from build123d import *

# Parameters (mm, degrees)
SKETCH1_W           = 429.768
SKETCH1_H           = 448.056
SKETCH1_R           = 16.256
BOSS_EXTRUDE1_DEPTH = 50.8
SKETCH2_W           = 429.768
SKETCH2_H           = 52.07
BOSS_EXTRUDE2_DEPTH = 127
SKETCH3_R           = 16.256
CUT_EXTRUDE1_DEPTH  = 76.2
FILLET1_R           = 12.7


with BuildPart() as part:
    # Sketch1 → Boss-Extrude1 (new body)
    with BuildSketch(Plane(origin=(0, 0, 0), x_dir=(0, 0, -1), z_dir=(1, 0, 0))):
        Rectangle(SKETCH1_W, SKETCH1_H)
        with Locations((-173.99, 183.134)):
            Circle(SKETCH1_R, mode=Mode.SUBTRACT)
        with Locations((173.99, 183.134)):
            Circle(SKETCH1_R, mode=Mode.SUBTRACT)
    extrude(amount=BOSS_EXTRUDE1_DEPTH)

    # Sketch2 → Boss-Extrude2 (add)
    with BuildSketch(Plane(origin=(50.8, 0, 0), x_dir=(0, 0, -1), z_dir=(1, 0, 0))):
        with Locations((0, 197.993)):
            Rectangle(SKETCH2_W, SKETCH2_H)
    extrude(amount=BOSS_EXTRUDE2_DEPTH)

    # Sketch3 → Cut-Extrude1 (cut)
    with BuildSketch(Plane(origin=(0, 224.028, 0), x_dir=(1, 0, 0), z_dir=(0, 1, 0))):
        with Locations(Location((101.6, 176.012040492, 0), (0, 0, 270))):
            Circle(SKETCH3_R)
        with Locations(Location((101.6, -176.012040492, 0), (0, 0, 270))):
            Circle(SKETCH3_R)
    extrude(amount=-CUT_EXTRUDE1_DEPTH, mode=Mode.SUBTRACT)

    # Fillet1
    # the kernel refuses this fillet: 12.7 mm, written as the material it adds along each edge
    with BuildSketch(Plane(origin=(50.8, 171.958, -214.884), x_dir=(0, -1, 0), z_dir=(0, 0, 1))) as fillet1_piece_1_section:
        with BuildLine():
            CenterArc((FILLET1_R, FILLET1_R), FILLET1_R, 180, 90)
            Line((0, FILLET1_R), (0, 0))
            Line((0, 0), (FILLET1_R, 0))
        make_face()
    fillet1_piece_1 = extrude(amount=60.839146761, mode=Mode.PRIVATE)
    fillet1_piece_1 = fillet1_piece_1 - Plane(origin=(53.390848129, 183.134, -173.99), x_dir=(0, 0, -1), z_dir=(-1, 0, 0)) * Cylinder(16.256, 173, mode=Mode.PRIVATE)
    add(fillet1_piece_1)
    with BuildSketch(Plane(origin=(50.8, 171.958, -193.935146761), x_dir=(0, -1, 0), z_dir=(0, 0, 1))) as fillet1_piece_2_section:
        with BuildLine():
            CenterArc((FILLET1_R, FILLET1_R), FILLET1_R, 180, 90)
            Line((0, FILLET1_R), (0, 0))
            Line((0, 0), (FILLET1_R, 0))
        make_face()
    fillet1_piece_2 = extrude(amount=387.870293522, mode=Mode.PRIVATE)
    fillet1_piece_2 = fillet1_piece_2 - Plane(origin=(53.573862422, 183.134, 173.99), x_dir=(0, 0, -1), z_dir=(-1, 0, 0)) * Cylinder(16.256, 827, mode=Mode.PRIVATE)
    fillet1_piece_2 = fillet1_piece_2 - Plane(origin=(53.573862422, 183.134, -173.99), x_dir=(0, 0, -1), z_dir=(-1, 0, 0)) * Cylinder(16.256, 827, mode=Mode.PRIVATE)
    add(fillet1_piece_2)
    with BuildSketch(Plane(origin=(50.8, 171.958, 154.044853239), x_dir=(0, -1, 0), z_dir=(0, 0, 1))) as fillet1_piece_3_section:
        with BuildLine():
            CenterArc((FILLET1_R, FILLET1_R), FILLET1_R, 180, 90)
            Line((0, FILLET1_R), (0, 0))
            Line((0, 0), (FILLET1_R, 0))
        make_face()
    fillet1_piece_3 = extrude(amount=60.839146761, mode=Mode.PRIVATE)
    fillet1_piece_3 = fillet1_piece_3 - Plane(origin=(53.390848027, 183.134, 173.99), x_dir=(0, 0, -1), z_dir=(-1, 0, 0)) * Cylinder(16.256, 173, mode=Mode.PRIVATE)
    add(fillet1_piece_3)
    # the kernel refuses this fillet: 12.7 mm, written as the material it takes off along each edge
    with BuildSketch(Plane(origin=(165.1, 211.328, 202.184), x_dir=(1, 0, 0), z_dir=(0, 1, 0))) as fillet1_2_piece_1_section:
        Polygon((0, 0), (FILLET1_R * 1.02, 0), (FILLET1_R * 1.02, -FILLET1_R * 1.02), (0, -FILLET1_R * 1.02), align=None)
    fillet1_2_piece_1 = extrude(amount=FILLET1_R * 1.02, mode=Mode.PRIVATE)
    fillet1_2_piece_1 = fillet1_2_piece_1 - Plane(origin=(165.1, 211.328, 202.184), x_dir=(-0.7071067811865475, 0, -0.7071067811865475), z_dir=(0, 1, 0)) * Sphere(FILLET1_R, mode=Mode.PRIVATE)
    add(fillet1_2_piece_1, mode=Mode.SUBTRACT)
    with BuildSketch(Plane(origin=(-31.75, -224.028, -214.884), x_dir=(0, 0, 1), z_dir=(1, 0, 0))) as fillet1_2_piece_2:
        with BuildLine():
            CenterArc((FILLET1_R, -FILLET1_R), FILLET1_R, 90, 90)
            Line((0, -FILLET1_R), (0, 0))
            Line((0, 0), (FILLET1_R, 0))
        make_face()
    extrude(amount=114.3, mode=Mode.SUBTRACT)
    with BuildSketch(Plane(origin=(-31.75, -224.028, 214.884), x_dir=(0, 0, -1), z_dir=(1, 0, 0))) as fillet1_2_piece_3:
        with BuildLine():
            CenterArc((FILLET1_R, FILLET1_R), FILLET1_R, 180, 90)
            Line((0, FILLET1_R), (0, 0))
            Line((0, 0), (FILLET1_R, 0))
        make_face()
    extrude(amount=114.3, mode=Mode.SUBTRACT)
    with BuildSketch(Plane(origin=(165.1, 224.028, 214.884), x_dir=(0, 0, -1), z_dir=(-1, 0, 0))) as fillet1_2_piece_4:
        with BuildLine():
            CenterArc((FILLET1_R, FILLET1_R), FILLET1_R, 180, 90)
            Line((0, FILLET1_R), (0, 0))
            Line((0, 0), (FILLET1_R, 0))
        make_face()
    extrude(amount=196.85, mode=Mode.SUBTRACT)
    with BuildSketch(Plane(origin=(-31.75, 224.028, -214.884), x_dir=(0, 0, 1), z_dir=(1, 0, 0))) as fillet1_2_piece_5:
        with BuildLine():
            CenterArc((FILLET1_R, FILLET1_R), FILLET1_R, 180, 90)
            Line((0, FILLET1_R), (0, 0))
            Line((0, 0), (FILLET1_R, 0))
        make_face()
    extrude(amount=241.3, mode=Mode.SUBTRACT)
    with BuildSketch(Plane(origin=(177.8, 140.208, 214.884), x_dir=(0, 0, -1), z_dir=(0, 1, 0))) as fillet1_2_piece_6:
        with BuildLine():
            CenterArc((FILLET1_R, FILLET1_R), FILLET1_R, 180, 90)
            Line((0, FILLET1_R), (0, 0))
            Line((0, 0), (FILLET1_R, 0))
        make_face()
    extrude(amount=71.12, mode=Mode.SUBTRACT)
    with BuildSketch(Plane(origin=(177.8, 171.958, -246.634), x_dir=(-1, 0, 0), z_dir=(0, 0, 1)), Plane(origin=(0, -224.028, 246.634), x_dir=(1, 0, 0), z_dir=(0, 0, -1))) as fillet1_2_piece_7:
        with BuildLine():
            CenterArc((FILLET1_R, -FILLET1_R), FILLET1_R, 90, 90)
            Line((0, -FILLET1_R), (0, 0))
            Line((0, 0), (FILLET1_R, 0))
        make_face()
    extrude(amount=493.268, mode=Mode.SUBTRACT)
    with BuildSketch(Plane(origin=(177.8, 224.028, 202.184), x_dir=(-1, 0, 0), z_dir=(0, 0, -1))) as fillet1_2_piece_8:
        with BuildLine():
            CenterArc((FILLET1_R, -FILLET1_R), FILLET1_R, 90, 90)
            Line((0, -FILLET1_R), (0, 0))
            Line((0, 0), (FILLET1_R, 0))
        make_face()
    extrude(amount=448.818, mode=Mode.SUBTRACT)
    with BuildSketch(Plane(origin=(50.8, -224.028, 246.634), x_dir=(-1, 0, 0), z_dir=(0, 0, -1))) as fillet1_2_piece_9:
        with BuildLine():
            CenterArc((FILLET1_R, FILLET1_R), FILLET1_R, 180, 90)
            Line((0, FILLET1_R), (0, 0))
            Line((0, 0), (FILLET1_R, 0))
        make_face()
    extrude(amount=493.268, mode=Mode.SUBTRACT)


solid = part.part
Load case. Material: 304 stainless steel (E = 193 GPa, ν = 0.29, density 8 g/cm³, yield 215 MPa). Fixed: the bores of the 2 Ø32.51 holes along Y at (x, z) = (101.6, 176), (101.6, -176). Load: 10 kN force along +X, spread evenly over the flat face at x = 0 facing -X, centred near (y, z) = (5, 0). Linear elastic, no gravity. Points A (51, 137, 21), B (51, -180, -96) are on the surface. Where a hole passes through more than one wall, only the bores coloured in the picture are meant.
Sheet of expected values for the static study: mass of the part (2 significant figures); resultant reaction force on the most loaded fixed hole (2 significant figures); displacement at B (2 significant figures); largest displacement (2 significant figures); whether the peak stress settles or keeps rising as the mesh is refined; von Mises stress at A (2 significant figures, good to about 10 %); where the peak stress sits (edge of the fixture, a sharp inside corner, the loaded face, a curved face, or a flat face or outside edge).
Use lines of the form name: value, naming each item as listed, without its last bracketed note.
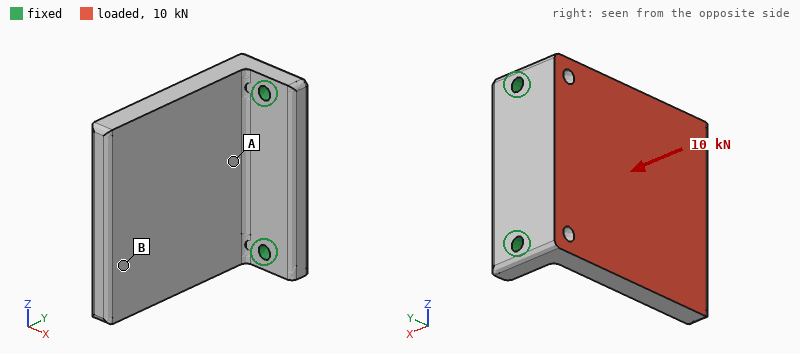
mass of the part: 99 kg
resultant reaction force on the most loaded fixed hole: 5.2 kN
displacement at B: 0.15 mm
largest displacement: 0.17 mm
whether the peak stress settles or keeps rising as the mesh is refined: keeps rising
von Mises stress at A: 7.1 MPa
where the peak stress sits: a sharp inside corner
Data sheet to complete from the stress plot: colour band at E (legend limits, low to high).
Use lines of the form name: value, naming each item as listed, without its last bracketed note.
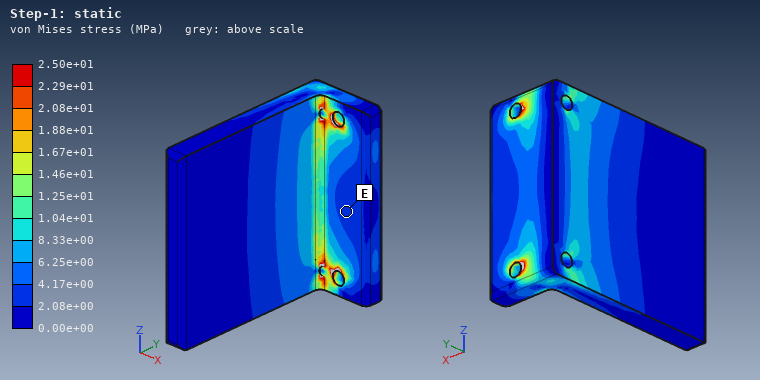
colour band at E: 2.08e+00 to 4.17e+00 MPa
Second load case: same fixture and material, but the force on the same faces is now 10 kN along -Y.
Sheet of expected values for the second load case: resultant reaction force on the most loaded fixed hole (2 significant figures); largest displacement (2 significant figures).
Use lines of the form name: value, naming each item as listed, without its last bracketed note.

resultant reaction force on the most loaded fixed hole: 5.0 kN
largest displacement: 48 µm
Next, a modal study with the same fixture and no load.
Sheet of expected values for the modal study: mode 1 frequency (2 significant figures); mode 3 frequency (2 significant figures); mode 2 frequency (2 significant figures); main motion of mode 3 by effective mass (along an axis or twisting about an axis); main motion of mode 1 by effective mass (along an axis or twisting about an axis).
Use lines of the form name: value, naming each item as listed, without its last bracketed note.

mode 1 frequency: 170 Hz
mode 3 frequency: 710 Hz
mode 2 frequency: 470 Hz
main motion of mode 3 by effective mass: along Z
main motion of mode 1 by effective mass: along X
